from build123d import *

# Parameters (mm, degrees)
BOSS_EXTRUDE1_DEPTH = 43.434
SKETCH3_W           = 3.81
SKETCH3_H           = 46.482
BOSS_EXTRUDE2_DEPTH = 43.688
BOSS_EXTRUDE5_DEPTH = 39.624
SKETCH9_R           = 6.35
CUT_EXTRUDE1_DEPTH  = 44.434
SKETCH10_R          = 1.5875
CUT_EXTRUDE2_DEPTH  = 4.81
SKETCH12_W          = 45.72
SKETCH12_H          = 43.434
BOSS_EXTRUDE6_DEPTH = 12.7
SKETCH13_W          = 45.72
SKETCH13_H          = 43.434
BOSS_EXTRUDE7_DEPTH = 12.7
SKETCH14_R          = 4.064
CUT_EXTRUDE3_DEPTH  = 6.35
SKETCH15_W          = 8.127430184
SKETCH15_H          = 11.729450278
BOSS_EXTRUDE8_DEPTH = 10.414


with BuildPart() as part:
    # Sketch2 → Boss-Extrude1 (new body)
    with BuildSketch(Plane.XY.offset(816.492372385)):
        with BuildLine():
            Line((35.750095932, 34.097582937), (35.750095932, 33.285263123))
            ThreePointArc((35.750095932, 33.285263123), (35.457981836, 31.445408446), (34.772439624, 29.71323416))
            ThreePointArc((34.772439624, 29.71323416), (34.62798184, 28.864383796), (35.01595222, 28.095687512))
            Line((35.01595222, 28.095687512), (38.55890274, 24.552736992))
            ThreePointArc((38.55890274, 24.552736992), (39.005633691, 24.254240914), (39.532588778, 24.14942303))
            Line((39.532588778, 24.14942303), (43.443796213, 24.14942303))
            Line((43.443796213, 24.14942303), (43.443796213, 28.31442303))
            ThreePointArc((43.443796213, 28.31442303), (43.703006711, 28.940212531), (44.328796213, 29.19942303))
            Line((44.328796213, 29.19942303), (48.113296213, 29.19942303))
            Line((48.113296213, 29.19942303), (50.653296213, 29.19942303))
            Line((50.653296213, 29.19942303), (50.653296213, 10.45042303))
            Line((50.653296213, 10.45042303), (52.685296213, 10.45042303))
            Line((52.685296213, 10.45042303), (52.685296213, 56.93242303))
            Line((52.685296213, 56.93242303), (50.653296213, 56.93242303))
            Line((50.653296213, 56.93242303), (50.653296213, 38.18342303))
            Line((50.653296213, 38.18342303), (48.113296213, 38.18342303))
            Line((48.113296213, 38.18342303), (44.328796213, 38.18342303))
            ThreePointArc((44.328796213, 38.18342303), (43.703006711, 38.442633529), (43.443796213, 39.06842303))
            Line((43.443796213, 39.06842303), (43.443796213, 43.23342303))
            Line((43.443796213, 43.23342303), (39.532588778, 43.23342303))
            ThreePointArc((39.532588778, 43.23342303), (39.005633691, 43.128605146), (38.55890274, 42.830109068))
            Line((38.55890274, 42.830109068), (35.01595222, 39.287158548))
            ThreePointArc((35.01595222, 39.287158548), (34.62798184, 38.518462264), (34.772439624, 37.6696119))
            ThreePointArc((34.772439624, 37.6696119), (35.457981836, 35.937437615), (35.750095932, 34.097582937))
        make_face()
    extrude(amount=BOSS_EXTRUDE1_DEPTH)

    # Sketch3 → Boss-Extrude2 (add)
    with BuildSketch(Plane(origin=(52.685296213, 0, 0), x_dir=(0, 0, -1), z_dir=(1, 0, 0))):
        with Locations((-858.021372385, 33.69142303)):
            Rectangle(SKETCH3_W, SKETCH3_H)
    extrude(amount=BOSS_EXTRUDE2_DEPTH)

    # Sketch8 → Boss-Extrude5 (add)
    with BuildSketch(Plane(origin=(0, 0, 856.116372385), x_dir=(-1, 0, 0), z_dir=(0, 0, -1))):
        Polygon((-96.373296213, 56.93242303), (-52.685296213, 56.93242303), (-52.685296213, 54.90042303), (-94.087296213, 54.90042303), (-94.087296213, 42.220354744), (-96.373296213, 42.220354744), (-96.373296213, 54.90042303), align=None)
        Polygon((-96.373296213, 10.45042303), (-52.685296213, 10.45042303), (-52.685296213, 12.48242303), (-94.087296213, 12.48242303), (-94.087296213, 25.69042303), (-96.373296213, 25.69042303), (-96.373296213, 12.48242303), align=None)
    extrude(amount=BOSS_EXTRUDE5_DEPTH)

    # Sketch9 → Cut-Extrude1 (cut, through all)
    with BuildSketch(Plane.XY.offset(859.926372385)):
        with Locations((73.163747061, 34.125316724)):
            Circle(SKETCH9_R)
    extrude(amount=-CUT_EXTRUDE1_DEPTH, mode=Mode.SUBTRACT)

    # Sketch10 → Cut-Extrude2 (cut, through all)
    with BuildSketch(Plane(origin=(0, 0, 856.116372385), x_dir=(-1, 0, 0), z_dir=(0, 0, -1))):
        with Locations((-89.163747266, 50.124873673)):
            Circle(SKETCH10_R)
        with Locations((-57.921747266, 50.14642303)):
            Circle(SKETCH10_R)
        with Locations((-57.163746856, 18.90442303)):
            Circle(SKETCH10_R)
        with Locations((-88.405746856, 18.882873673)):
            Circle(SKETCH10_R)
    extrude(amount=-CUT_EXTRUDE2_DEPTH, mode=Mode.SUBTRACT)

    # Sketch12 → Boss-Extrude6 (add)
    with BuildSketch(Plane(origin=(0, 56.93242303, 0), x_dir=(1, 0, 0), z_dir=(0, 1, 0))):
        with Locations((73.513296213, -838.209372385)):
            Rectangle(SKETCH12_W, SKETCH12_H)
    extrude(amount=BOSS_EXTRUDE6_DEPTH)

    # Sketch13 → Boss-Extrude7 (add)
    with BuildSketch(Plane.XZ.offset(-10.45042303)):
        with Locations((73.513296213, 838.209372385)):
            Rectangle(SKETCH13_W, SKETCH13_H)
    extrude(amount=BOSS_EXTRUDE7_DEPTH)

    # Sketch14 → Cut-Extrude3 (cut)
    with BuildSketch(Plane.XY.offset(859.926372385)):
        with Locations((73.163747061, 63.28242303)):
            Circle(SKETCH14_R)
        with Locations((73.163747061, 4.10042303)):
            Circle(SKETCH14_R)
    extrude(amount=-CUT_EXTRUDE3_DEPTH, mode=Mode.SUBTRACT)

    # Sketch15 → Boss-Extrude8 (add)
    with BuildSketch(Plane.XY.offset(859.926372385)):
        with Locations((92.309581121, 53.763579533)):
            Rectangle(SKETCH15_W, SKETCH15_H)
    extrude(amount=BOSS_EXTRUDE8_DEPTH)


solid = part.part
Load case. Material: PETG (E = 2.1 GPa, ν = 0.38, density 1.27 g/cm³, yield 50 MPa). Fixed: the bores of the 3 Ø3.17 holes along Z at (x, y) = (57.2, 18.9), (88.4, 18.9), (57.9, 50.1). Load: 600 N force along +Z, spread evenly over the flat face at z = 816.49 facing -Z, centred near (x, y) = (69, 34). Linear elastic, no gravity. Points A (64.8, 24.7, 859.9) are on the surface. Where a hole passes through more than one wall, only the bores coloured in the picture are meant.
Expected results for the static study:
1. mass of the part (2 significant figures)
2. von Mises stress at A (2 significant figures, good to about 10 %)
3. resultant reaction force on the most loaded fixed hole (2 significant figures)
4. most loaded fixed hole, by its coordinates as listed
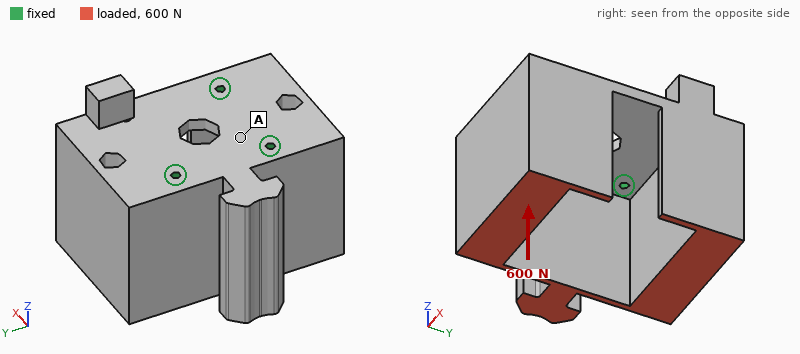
100 g
1.9 MPa
290 N
(57.9, 50.1)
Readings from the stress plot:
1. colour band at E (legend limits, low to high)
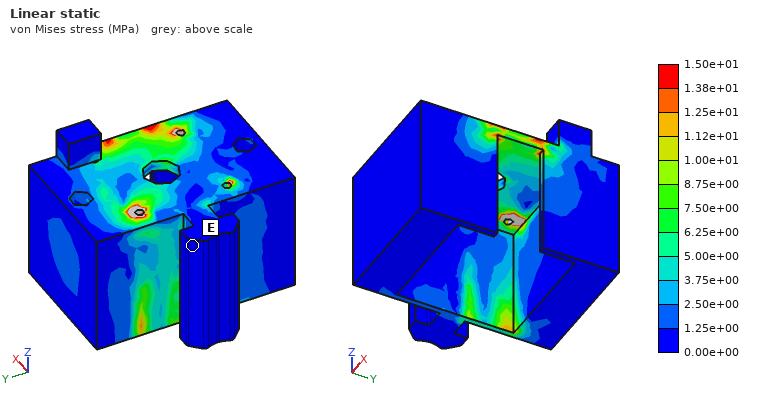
0.00e+00 to 1.25e+00 MPa
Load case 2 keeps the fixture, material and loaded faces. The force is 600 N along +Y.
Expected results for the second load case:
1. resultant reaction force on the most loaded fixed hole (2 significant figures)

690 N
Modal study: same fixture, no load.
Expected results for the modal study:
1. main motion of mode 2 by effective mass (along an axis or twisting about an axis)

along Y
